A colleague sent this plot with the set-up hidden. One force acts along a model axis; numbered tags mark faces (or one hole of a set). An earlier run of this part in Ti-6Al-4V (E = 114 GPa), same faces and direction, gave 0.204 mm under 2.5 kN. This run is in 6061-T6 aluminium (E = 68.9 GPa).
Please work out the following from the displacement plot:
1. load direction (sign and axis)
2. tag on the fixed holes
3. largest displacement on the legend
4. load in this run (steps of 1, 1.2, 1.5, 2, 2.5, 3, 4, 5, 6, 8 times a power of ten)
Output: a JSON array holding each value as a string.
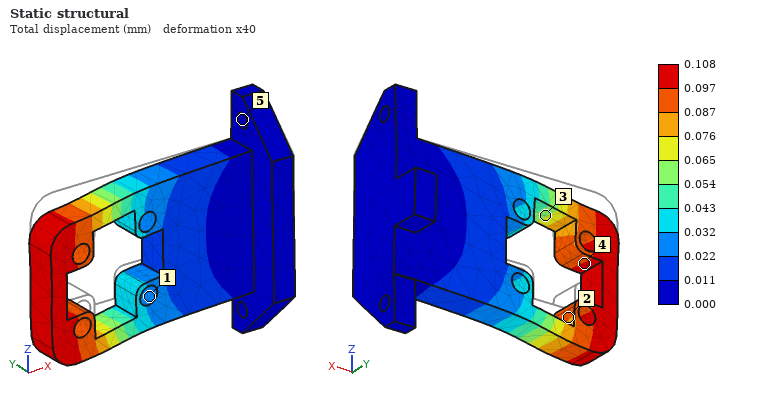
["-Z", "5", "0.108 mm", "800 N"]
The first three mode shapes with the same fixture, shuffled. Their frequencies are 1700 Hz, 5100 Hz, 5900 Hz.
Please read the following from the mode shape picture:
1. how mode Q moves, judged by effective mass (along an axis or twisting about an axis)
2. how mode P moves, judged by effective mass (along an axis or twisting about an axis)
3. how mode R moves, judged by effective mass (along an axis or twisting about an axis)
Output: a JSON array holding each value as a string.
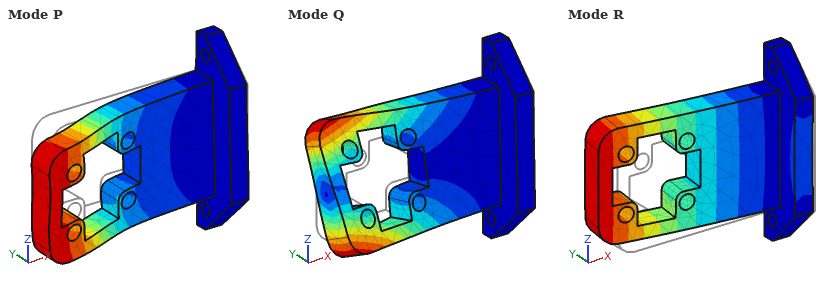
["twisting about X", "along Z", "along Y"]
